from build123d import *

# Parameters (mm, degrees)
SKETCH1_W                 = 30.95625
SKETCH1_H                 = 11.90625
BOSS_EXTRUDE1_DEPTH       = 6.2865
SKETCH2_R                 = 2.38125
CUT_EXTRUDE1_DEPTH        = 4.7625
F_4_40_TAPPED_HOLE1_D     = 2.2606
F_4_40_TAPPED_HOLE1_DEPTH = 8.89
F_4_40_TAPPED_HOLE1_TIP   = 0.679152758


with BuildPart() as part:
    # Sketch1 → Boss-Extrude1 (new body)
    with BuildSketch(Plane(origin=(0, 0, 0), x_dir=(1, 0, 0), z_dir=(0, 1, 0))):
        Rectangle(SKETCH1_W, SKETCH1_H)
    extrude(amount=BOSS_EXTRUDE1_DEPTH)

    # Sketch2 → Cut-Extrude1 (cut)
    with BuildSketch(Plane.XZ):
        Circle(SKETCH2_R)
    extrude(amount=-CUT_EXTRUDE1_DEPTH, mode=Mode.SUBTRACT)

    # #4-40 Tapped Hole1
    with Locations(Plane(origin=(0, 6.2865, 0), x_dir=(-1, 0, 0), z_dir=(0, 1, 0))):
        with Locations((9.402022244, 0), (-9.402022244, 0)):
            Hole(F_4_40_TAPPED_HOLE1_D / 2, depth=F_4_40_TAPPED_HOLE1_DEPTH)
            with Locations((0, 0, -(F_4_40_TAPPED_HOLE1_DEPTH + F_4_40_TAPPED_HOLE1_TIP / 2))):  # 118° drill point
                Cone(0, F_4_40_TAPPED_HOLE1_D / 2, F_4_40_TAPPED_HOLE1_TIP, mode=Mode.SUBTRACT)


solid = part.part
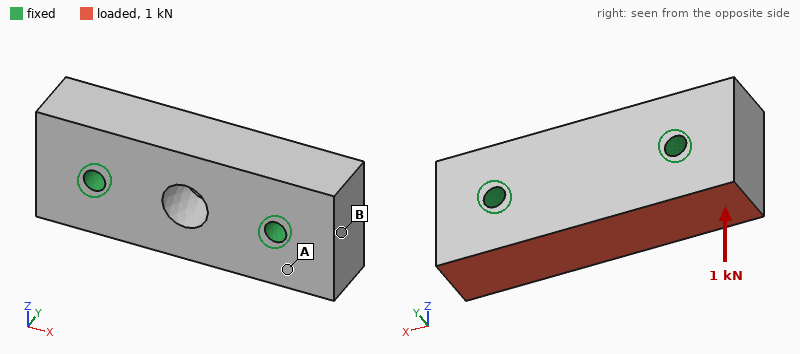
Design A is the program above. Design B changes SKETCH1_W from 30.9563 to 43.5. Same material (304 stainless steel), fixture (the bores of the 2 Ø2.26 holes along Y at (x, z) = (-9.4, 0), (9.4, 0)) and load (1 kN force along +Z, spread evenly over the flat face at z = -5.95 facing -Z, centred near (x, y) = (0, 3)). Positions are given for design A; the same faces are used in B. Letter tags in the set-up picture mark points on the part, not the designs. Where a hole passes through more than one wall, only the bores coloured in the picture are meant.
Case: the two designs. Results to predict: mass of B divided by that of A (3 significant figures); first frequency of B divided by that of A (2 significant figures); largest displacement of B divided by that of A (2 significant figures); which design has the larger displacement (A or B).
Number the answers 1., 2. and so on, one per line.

1. 1.43
2. 0.49
3. 2.7
4. B
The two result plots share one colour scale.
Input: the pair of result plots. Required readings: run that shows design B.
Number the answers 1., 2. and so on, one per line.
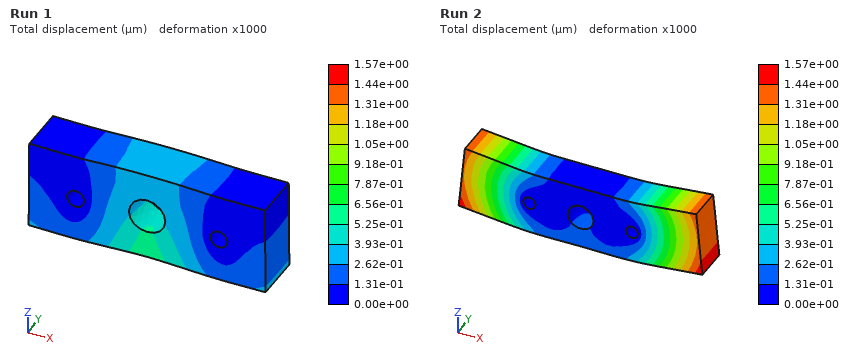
1. Run 2
